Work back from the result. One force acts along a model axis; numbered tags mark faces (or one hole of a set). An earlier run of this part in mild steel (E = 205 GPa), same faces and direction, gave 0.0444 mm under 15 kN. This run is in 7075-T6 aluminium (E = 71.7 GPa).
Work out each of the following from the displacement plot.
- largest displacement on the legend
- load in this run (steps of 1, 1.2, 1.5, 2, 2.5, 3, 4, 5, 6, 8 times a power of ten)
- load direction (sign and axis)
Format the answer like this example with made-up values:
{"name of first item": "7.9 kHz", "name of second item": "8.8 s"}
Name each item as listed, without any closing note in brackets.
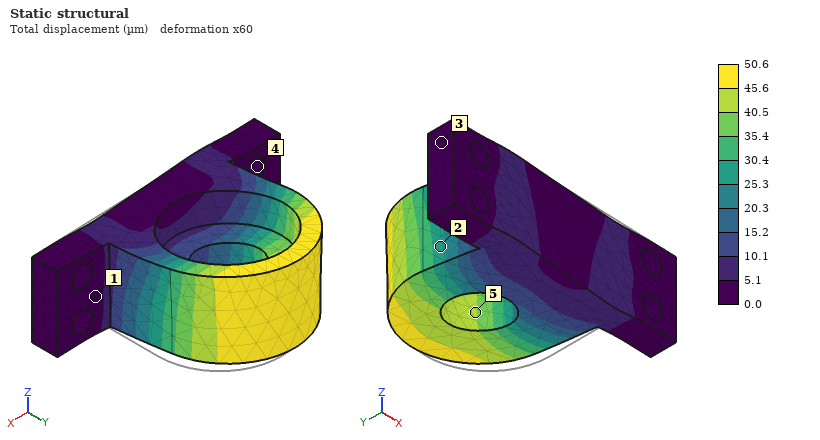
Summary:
{"largest displacement on the legend": "50.6 µm", "load in this run": "6 kN", "load direction": "-X"}
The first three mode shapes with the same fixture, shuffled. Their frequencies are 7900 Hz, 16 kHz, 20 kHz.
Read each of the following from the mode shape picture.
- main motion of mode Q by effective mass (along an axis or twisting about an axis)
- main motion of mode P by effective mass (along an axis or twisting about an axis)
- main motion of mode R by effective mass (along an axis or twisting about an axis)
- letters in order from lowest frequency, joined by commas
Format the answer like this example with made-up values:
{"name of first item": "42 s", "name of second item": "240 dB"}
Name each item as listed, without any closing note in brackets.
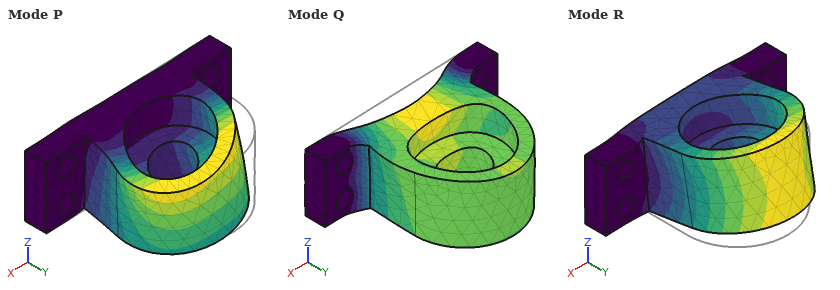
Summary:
{"main motion of mode Q by effective mass": "along Y", "main motion of mode P by effective mass": "along X", "main motion of mode R by effective mass": "along Z", "letters in order from lowest frequency, joined by commas": "R, P, Q"}
